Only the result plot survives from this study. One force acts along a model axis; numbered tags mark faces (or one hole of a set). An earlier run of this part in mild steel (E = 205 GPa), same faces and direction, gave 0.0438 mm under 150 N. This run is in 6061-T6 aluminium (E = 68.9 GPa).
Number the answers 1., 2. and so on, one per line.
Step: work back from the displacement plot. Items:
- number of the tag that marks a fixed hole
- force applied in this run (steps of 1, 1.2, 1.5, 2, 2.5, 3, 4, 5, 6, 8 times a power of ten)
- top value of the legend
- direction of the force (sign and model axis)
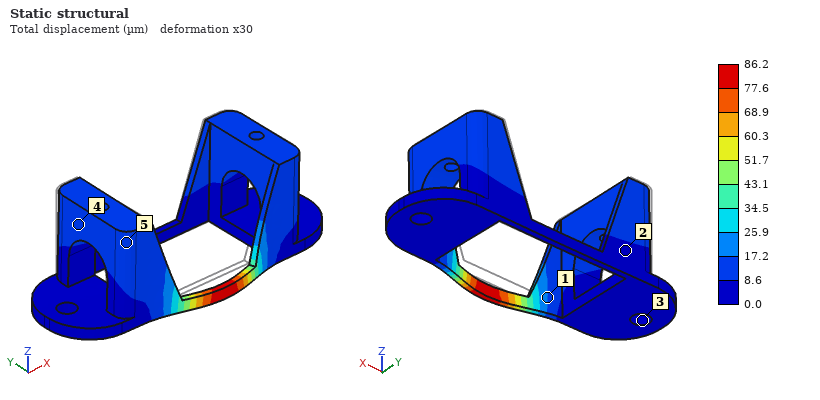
1. 3
2. 100 N
3. 86.2 µm
4. -Y
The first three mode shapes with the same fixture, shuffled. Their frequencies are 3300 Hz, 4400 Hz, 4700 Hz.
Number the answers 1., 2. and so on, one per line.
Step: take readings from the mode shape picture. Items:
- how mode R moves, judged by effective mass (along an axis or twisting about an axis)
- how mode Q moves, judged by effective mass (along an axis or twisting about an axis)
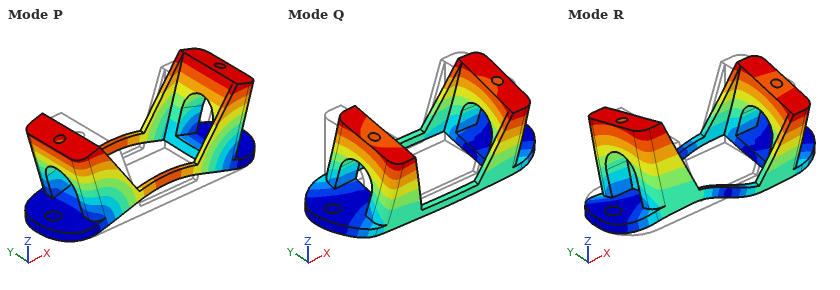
1. twisting about Z
2. along Y
